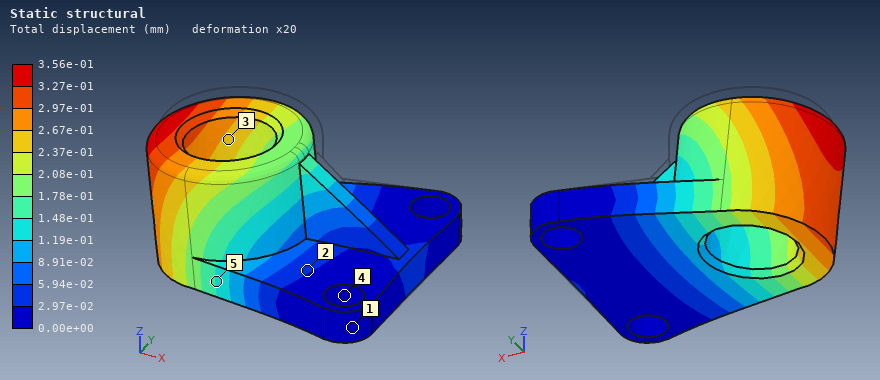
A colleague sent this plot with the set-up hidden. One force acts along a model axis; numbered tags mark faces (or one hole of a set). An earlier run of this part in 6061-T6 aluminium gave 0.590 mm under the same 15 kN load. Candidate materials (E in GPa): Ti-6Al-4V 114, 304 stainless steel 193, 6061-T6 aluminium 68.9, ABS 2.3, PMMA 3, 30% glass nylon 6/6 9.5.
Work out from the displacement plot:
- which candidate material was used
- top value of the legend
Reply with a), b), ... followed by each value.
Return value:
a) Ti-6Al-4V
b) 3.56e-01 mm
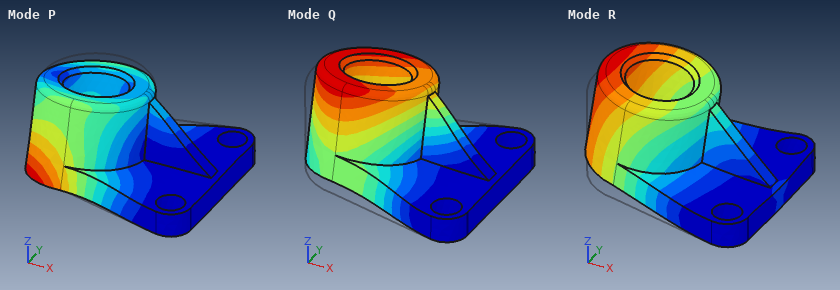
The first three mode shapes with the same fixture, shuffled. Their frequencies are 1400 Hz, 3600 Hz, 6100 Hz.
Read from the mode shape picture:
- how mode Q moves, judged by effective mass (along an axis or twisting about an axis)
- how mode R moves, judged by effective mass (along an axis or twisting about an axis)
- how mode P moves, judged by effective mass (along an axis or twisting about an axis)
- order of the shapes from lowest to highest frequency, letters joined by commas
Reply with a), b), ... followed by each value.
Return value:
a) along Y
b) along Z
c) along Y
d) R, Q, P
